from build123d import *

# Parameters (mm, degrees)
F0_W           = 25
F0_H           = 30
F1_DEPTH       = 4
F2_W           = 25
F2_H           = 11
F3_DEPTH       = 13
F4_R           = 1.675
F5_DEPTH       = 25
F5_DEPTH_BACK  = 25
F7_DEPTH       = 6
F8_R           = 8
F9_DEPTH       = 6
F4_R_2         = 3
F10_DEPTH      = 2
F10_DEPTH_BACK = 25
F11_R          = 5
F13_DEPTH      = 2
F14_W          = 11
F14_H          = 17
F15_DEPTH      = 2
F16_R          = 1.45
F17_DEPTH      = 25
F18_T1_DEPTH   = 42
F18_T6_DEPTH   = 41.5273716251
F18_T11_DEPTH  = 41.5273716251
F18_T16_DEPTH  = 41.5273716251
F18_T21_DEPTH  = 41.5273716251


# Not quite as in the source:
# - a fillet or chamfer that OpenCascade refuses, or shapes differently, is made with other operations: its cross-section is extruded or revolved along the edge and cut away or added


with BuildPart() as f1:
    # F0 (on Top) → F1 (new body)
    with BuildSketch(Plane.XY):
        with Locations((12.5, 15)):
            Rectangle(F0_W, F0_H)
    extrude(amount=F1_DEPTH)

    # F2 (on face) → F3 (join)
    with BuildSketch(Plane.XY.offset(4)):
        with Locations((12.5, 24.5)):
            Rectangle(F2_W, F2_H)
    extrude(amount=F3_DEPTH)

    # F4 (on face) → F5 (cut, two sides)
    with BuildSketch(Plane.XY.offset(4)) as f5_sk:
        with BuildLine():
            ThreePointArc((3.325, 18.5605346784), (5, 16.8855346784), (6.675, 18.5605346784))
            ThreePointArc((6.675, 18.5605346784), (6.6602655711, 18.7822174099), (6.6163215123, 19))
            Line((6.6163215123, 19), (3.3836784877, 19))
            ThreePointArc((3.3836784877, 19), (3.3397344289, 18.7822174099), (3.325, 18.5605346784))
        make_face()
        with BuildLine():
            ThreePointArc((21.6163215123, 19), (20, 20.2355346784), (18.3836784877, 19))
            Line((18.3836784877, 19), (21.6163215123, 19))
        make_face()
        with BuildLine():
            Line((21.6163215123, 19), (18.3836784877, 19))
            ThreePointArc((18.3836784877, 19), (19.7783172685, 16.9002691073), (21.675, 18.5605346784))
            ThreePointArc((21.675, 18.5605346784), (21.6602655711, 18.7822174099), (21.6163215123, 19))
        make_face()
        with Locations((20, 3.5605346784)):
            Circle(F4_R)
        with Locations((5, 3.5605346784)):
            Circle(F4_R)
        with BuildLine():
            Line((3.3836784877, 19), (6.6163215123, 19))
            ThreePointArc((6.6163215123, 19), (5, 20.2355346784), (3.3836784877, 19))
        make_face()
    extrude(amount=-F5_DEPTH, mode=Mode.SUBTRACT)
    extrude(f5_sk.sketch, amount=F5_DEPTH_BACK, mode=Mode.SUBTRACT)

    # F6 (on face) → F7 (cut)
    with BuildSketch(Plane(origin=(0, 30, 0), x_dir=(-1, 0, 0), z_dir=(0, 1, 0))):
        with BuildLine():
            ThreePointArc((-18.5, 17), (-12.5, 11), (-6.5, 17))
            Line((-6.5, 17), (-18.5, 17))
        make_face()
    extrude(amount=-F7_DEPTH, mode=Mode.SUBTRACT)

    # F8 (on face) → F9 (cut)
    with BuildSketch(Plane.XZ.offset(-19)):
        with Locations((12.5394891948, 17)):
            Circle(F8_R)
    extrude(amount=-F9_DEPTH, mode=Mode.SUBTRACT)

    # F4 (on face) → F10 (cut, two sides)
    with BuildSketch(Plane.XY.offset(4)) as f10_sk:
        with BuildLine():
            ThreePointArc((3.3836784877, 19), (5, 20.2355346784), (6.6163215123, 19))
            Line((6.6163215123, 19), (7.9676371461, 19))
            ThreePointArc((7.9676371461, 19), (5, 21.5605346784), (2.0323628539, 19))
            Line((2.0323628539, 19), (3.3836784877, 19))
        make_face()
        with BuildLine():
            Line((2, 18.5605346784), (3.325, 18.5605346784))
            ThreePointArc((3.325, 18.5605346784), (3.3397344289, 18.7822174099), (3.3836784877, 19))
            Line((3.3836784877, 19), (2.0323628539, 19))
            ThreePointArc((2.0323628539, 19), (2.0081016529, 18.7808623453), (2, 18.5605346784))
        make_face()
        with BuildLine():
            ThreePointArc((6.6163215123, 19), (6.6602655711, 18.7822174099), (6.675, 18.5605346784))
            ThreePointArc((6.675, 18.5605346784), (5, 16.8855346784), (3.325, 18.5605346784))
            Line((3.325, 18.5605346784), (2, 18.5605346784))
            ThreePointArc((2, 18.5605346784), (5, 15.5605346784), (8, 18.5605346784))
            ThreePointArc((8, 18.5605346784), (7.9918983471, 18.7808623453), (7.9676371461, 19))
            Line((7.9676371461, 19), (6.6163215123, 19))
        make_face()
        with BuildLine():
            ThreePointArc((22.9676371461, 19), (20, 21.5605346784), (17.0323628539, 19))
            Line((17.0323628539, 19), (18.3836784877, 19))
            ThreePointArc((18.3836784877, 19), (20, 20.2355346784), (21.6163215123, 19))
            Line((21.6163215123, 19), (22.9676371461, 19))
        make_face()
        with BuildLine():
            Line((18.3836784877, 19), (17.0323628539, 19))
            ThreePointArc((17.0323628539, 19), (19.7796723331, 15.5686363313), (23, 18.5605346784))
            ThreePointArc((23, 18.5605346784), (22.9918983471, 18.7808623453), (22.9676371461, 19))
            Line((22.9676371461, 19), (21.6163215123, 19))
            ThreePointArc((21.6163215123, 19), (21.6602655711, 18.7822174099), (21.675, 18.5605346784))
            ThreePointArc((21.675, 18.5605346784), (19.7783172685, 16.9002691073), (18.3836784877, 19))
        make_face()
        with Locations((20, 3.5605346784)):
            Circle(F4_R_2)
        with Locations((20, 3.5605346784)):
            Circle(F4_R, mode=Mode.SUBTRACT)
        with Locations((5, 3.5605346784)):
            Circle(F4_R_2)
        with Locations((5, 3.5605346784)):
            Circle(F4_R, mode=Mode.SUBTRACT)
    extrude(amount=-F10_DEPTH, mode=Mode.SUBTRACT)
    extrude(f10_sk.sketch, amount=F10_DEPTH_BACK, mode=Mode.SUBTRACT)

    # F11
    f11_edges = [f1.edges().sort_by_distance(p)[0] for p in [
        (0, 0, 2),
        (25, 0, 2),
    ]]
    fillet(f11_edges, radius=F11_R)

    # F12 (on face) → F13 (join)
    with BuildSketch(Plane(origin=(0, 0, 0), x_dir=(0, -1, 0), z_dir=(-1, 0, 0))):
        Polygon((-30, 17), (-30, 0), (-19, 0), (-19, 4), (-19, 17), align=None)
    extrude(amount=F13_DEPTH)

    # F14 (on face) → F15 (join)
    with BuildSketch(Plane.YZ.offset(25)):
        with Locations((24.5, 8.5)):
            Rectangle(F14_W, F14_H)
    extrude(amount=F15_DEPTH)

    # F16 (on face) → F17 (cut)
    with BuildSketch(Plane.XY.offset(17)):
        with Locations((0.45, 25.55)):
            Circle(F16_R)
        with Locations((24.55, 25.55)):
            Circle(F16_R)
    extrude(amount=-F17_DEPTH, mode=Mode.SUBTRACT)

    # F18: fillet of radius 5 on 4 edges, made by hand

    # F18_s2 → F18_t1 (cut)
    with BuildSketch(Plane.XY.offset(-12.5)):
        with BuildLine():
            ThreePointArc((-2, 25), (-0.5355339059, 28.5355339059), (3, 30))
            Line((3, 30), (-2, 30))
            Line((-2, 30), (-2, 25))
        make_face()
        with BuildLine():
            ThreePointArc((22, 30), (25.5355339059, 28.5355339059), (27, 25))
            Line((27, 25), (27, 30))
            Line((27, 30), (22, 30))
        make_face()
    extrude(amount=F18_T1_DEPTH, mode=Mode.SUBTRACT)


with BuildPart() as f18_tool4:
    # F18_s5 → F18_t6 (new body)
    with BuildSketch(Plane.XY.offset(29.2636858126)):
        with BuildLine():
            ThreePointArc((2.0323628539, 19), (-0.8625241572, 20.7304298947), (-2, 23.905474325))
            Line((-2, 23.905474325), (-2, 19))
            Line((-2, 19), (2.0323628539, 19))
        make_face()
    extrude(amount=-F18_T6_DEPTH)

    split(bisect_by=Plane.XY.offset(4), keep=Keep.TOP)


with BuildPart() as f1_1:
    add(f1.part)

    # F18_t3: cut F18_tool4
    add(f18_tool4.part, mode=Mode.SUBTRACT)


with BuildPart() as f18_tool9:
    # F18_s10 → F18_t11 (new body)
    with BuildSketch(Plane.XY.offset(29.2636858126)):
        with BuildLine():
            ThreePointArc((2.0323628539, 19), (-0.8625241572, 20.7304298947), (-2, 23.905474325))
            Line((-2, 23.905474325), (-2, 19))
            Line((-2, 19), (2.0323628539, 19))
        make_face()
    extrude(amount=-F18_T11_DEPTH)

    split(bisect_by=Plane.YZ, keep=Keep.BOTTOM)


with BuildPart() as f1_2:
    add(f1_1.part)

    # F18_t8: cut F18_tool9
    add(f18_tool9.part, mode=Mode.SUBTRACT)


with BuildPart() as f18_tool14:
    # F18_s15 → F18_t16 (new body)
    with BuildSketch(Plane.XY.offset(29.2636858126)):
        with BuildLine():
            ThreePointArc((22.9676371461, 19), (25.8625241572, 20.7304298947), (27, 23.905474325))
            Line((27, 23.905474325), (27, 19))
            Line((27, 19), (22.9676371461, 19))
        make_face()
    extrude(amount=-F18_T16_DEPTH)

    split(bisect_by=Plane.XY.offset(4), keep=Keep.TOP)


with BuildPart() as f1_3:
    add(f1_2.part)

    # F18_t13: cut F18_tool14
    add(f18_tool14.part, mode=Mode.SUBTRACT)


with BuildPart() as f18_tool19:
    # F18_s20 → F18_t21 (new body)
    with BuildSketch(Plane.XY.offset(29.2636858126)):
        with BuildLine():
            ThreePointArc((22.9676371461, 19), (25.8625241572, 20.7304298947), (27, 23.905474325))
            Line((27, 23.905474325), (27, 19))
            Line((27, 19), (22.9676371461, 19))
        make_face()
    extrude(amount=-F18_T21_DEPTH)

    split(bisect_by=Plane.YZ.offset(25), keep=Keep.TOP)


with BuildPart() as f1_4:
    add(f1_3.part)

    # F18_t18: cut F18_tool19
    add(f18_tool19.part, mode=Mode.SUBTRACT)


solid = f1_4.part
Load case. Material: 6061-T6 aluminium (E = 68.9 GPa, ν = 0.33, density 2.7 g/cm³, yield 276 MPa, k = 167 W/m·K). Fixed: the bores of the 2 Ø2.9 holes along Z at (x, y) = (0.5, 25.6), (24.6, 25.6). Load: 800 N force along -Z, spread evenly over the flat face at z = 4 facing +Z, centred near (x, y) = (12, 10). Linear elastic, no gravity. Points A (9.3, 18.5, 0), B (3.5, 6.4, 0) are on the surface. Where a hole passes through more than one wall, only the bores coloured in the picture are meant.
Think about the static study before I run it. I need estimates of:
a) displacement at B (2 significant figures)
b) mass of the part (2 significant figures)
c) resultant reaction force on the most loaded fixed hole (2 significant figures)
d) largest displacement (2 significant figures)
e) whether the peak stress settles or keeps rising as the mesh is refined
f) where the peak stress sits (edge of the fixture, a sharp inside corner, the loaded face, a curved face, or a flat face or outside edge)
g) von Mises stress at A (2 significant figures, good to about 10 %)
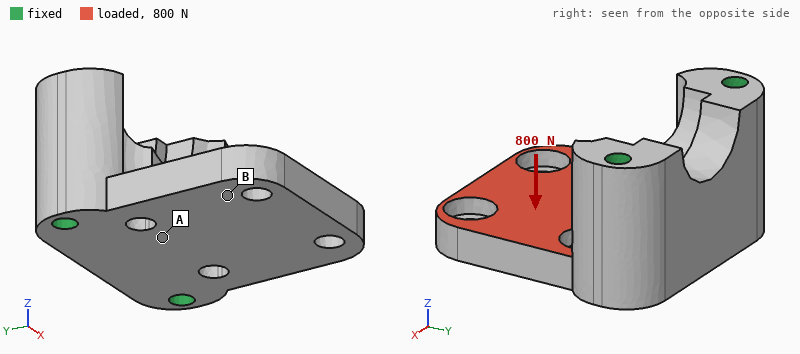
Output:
0.10 mm
14 g
400 N
0.16 mm
keeps rising
a sharp inside corner
120 MPa
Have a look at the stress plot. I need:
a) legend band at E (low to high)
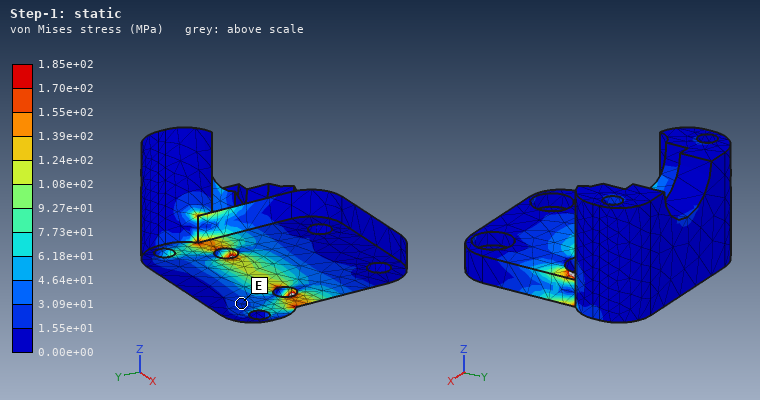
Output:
1.55e+01 to 3.09e+01 MPa
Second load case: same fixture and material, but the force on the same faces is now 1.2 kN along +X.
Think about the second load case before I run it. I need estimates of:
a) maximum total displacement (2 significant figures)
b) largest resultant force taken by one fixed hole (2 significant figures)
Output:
32 µm
980 N
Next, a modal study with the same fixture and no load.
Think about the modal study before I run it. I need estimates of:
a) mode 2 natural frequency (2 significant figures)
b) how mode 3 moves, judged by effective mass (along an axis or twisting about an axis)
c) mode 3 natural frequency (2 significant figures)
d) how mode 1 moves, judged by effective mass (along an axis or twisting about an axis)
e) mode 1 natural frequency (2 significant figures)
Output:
15 kHz
along X
23 kHz
along Z
6800 Hz
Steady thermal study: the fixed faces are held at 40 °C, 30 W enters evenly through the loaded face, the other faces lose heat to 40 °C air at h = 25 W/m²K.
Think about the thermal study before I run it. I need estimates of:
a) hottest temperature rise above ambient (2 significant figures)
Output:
32 K
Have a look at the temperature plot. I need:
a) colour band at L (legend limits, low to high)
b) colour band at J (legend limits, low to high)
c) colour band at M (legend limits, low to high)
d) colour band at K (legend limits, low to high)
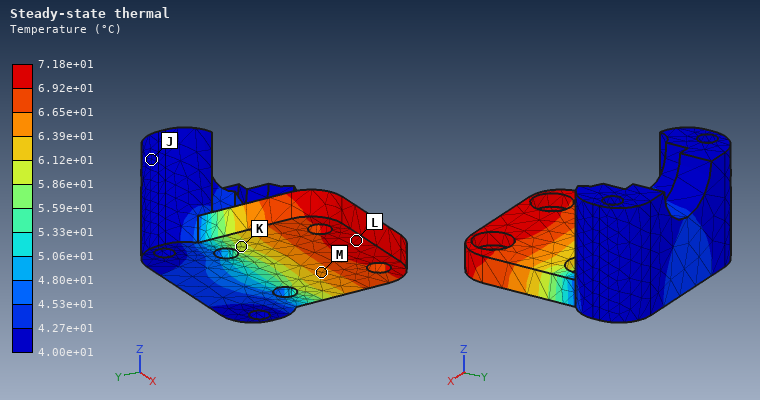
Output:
6.92e+01 to 7.18e+01 °C
4.00e+01 to 4.27e+01 °C
6.39e+01 to 6.65e+01 °C
5.86e+01 to 6.12e+01 °C
